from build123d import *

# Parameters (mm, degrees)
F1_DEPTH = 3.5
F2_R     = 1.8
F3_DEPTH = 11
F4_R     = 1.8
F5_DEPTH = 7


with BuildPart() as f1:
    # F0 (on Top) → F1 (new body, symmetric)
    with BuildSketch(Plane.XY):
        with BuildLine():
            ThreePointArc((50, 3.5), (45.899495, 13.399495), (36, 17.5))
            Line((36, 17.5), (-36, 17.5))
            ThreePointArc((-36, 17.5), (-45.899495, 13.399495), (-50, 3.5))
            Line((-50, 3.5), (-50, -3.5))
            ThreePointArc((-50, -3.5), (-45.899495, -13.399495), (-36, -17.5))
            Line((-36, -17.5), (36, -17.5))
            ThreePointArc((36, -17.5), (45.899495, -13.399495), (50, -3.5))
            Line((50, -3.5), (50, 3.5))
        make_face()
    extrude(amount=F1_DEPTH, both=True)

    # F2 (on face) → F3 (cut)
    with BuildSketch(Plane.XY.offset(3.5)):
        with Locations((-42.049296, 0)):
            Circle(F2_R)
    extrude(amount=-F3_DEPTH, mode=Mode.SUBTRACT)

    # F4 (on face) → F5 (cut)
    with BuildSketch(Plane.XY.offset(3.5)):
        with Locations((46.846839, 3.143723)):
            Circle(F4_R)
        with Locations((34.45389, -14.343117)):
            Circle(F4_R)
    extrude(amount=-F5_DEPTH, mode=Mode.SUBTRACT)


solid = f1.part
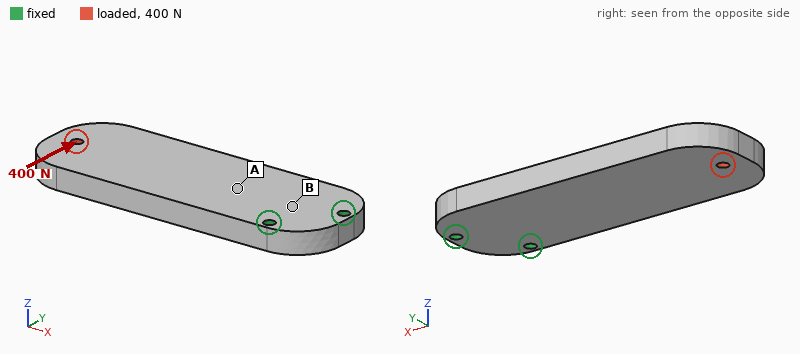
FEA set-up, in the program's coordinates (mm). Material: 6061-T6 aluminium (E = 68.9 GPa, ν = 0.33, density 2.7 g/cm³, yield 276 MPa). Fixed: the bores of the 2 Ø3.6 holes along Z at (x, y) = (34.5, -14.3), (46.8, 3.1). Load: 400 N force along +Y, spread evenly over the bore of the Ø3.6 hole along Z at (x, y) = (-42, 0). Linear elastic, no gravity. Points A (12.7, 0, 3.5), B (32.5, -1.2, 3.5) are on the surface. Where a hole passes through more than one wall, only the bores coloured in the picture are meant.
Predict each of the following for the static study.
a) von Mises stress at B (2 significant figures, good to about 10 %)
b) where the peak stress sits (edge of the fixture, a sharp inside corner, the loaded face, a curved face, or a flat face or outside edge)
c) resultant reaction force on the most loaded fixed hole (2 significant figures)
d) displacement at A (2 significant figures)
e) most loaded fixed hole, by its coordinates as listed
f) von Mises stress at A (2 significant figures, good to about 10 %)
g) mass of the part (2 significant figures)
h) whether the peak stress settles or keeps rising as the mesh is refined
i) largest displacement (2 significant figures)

8.8 MPa
edge of the fixture
1.5 kN
11 µm
(34.5, -14.3)
4.4 MPa
62 g
keeps rising
65 µm
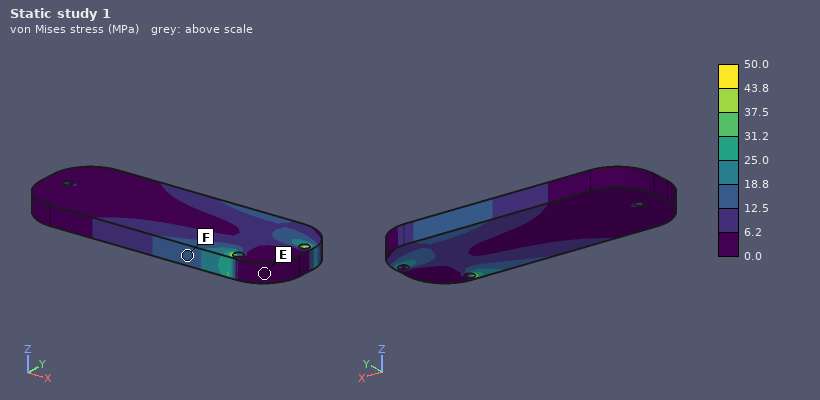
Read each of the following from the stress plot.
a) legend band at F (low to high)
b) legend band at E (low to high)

12.5 to 18.8 MPa
0.0 to 6.2 MPa
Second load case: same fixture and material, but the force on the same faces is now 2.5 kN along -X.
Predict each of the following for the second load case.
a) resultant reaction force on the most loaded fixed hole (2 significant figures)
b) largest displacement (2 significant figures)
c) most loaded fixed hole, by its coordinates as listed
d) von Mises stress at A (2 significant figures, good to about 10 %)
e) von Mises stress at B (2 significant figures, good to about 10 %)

1.7 kN
25 µm
(46.8, 3.1)
10 MPa
13 MPa
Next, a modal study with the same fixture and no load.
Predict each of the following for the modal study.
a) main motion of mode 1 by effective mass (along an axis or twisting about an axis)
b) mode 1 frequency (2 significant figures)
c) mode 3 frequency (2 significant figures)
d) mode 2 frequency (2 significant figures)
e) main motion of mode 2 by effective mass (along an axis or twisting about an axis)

along Z
740 Hz
3400 Hz
3000 Hz
along Y
